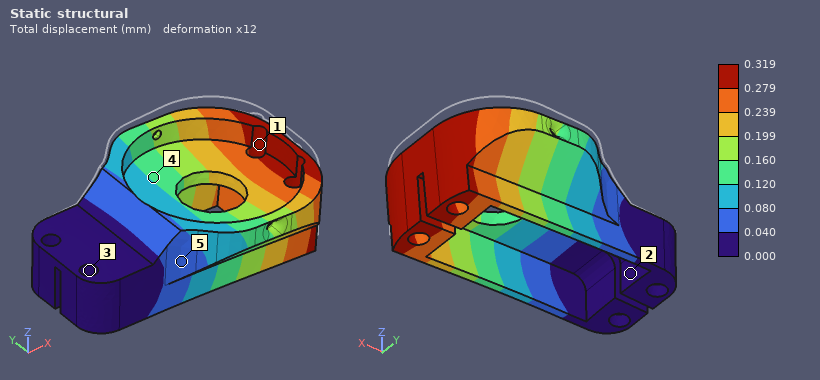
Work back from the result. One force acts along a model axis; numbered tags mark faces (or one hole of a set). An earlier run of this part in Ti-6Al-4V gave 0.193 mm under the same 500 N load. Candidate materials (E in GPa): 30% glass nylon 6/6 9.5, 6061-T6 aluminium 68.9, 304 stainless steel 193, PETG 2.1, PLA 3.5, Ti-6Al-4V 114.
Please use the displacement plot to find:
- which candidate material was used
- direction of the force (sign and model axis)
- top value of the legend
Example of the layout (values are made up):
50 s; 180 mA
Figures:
6061-T6 aluminium; -Z; 0.319 mm
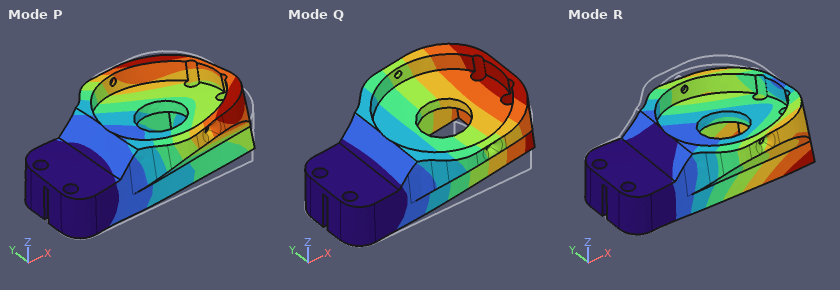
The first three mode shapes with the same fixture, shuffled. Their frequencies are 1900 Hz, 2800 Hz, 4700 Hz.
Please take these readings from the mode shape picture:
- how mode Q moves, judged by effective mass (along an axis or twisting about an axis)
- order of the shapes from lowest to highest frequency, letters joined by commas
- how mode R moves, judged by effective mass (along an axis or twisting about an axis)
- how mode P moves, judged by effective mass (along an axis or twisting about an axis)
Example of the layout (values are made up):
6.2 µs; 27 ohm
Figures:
along Z; Q, R, P; along Y; along Y
